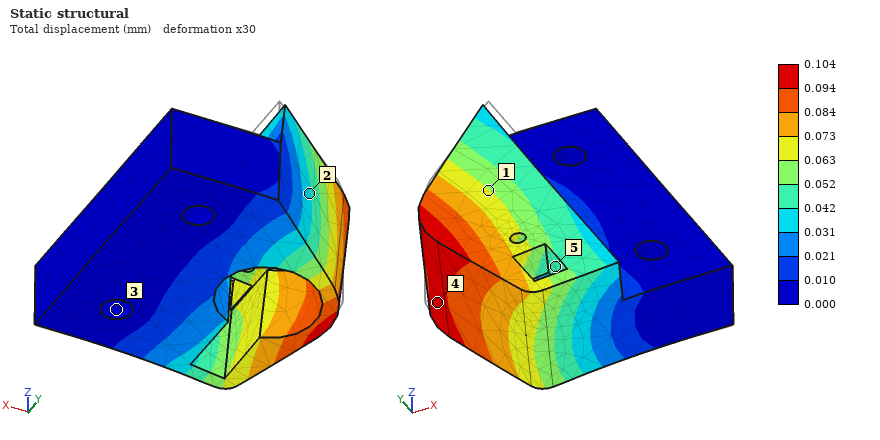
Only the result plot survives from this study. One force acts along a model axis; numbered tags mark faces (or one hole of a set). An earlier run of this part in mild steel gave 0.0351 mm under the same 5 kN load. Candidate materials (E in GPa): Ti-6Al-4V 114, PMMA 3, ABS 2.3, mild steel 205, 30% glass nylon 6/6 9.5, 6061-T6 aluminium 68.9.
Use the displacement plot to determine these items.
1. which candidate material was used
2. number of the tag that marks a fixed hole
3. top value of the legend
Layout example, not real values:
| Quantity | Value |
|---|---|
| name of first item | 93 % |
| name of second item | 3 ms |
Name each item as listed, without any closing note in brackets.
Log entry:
| Quantity | Value |
|---|---|
| which candidate material was used | 6061-T6 aluminium |
| number of the tag that marks a fixed hole | 3 |
| top value of the legend | 0.104 mm |
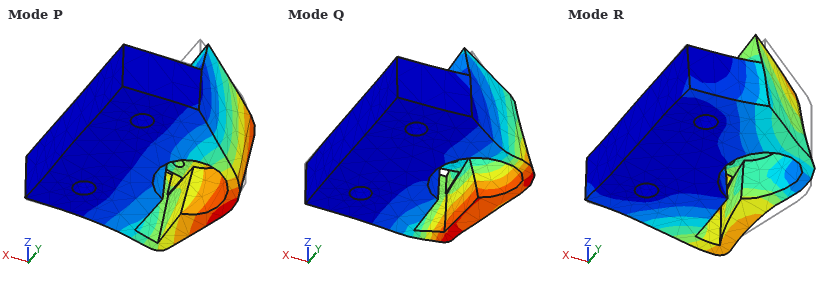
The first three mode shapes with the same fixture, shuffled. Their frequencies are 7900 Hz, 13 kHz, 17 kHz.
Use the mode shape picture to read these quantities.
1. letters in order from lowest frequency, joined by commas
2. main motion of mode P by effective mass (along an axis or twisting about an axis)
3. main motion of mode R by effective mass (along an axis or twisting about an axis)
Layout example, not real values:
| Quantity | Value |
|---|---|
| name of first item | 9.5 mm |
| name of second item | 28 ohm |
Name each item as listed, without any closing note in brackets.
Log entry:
| Quantity | Value |
|---|---|
| letters in order from lowest frequency, joined by commas | P, Q, R |
| main motion of mode P by effective mass | along Z |
| main motion of mode R by effective mass | along Y |
